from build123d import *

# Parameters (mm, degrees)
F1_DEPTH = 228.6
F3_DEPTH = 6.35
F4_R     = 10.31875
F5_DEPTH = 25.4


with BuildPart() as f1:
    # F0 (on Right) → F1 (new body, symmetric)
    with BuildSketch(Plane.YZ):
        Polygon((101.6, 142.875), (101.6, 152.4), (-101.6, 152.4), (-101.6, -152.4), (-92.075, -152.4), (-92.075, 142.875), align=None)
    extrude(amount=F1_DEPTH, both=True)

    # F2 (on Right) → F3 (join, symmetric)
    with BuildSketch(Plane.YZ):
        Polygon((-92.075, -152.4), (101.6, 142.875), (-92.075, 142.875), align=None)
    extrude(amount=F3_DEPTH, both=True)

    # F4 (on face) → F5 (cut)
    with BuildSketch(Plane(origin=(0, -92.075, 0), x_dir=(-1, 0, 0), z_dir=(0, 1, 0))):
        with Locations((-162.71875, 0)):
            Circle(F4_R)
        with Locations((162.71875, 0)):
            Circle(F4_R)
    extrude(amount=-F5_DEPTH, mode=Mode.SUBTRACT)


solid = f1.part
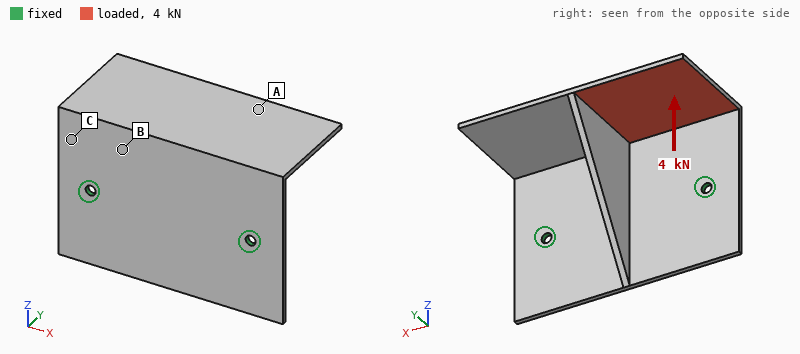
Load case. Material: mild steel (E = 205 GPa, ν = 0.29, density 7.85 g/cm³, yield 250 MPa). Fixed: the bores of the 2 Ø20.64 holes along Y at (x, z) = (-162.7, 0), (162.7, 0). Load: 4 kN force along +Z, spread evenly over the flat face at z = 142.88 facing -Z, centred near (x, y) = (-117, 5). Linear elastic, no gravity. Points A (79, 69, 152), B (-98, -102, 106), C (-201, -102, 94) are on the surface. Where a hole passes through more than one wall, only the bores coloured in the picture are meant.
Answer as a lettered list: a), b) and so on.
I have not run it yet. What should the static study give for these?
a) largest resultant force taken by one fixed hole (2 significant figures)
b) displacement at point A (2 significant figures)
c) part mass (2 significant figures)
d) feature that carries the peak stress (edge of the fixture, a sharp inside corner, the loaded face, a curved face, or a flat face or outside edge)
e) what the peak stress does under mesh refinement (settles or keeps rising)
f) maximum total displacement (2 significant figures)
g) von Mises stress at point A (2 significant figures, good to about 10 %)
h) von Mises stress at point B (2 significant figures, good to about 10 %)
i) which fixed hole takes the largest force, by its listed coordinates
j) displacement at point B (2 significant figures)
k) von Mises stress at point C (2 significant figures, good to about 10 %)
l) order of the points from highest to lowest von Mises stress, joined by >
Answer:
a) 3.4 kN
b) 0.64 mm
c) 20 kg
d) edge of the fixture
e) keeps rising
f) 1.6 mm
g) 8.4 MPa
h) 22 MPa
i) (-162.7, 0)
j) 0.30 mm
k) 34 MPa
l) C > B > A
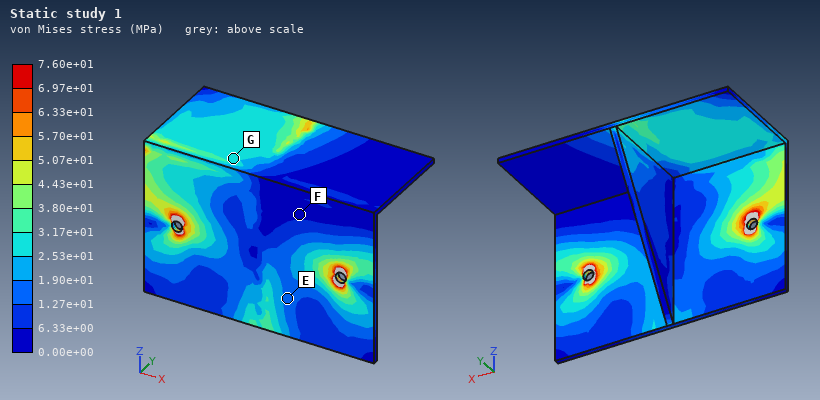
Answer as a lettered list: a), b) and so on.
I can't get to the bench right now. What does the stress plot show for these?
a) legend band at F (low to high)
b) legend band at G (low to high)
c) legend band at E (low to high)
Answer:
a) 0.00e+00 to 6.33e+00 MPa
b) 2.53e+01 to 3.17e+01 MPa
c) 1.27e+01 to 1.90e+01 MPa
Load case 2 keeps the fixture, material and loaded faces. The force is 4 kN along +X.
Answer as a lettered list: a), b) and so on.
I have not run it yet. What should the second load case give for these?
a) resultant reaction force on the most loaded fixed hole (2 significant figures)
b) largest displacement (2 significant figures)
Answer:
a) 2.9 kN
b) 0.41 mm
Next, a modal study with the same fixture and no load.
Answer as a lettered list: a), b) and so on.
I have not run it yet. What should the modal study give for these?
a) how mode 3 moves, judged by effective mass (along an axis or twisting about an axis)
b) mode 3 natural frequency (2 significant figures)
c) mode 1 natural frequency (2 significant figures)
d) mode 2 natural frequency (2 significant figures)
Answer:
a) along Y
b) 260 Hz
c) 100 Hz
d) 180 Hz
